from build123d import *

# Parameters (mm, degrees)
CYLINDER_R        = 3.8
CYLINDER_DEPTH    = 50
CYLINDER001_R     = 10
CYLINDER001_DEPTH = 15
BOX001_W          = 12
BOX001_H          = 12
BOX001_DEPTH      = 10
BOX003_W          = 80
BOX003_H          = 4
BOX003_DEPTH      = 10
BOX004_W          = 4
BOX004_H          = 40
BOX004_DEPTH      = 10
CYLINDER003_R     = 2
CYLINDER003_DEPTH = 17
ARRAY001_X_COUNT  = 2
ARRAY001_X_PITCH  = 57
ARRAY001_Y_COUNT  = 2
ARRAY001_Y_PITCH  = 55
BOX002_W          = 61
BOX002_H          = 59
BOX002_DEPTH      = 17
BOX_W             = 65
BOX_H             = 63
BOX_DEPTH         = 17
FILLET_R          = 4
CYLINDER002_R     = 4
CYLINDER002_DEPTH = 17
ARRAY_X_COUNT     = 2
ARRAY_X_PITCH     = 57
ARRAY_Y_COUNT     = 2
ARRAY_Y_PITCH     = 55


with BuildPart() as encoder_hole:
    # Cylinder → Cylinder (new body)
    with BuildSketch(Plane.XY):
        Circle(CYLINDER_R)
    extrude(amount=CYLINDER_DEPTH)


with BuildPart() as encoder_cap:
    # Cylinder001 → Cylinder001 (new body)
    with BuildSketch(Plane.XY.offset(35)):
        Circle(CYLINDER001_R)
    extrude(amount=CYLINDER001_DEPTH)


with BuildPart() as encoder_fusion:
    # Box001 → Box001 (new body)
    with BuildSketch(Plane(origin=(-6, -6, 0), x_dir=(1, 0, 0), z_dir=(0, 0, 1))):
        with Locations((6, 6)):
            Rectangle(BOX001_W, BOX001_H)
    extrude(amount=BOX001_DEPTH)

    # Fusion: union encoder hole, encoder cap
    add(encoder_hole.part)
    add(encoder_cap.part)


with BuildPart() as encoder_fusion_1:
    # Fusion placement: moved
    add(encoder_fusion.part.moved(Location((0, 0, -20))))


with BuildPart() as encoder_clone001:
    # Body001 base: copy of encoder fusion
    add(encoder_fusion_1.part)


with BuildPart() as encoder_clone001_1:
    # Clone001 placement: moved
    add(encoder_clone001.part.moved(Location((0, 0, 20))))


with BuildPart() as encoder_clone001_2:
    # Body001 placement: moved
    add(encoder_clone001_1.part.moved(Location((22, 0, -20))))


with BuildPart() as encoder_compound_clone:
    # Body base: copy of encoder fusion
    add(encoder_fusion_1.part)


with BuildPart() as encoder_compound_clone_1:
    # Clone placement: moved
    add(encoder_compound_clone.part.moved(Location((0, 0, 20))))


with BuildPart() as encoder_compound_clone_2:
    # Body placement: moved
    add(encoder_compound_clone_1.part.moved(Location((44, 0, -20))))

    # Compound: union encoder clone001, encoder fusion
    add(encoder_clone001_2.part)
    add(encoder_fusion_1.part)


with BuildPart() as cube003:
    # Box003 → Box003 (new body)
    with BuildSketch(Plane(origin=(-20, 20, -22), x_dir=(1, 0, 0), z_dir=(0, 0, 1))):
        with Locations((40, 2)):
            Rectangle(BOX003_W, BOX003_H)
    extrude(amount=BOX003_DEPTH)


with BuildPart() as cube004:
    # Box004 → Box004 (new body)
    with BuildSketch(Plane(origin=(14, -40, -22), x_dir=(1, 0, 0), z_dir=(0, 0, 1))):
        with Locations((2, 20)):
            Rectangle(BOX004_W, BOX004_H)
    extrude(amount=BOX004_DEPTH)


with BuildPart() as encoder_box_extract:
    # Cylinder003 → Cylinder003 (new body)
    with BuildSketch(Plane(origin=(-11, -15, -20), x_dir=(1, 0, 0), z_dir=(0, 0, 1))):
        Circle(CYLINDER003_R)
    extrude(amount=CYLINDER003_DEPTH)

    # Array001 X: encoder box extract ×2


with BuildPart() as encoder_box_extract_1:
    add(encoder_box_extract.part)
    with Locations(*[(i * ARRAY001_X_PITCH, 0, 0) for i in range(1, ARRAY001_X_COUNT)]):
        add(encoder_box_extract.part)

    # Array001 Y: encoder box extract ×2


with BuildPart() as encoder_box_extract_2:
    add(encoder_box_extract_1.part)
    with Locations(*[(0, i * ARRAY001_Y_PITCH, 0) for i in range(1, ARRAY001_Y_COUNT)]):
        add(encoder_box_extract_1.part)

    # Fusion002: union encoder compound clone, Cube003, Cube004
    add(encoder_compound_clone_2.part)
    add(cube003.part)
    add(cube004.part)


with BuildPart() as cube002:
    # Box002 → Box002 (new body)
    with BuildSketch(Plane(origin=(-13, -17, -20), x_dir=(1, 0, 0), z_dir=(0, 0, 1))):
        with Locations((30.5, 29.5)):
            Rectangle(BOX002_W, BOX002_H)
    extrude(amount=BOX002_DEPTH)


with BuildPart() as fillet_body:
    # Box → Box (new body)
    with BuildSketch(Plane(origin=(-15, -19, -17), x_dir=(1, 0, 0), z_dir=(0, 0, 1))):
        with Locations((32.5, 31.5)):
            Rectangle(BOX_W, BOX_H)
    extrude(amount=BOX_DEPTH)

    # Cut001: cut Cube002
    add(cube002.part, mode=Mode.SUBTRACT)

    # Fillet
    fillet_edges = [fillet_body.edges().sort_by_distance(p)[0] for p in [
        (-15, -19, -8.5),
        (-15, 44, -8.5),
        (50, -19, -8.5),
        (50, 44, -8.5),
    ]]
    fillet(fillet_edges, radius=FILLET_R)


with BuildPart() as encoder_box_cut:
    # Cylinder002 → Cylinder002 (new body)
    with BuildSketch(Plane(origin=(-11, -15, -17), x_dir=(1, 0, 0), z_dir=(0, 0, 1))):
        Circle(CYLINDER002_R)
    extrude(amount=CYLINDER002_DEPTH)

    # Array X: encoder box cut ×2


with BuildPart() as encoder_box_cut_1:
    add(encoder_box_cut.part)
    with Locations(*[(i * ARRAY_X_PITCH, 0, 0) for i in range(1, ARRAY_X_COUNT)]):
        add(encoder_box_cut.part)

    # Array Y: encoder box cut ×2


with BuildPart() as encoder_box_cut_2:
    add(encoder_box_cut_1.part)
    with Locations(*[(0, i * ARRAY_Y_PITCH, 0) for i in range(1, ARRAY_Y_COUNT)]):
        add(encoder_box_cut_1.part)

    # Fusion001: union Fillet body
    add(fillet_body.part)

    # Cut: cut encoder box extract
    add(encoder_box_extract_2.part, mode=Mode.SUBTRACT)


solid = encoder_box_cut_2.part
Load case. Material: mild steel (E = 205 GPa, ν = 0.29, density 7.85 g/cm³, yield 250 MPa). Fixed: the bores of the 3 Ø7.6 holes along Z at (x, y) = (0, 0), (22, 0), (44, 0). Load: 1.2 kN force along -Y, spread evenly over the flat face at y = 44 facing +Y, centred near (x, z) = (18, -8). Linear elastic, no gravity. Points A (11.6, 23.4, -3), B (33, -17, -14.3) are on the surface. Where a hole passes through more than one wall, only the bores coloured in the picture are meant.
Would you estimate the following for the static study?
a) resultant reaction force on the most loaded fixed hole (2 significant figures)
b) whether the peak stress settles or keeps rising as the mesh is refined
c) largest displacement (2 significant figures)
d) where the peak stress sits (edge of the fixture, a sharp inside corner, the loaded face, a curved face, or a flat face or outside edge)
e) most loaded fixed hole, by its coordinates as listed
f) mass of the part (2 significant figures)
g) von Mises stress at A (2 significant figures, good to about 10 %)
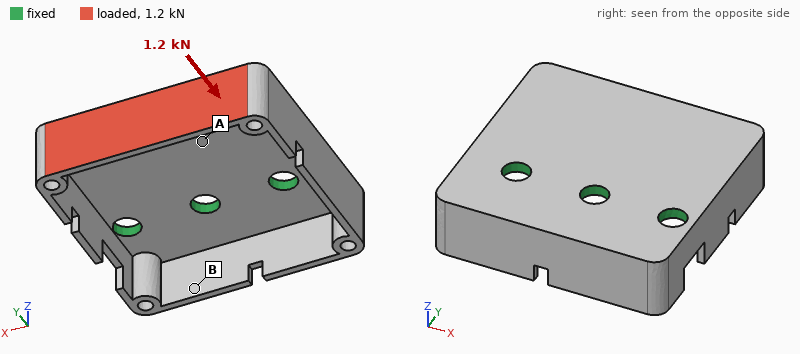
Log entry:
660 N
keeps rising
98 µm
edge of the fixture
(0, 0)
150 g
25 MPa
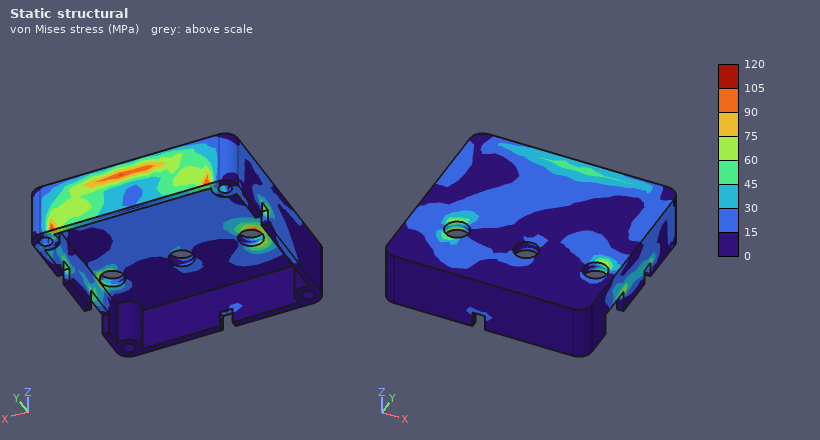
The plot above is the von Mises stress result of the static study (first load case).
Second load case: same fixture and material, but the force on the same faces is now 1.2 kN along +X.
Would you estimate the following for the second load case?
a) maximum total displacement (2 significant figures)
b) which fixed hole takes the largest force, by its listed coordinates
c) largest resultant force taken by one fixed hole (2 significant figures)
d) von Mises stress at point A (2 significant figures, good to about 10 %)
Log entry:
81 µm
(0, 0)
1.3 kN
40 MPa
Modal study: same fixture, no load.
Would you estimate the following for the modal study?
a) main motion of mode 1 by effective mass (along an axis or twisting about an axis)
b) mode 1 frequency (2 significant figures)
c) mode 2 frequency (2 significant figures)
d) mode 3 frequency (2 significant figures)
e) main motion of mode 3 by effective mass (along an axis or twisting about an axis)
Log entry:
along Z
1600 Hz
2300 Hz
5800 Hz
along Z
